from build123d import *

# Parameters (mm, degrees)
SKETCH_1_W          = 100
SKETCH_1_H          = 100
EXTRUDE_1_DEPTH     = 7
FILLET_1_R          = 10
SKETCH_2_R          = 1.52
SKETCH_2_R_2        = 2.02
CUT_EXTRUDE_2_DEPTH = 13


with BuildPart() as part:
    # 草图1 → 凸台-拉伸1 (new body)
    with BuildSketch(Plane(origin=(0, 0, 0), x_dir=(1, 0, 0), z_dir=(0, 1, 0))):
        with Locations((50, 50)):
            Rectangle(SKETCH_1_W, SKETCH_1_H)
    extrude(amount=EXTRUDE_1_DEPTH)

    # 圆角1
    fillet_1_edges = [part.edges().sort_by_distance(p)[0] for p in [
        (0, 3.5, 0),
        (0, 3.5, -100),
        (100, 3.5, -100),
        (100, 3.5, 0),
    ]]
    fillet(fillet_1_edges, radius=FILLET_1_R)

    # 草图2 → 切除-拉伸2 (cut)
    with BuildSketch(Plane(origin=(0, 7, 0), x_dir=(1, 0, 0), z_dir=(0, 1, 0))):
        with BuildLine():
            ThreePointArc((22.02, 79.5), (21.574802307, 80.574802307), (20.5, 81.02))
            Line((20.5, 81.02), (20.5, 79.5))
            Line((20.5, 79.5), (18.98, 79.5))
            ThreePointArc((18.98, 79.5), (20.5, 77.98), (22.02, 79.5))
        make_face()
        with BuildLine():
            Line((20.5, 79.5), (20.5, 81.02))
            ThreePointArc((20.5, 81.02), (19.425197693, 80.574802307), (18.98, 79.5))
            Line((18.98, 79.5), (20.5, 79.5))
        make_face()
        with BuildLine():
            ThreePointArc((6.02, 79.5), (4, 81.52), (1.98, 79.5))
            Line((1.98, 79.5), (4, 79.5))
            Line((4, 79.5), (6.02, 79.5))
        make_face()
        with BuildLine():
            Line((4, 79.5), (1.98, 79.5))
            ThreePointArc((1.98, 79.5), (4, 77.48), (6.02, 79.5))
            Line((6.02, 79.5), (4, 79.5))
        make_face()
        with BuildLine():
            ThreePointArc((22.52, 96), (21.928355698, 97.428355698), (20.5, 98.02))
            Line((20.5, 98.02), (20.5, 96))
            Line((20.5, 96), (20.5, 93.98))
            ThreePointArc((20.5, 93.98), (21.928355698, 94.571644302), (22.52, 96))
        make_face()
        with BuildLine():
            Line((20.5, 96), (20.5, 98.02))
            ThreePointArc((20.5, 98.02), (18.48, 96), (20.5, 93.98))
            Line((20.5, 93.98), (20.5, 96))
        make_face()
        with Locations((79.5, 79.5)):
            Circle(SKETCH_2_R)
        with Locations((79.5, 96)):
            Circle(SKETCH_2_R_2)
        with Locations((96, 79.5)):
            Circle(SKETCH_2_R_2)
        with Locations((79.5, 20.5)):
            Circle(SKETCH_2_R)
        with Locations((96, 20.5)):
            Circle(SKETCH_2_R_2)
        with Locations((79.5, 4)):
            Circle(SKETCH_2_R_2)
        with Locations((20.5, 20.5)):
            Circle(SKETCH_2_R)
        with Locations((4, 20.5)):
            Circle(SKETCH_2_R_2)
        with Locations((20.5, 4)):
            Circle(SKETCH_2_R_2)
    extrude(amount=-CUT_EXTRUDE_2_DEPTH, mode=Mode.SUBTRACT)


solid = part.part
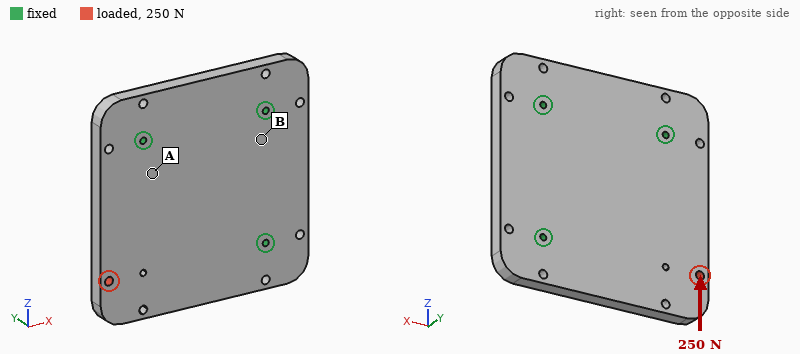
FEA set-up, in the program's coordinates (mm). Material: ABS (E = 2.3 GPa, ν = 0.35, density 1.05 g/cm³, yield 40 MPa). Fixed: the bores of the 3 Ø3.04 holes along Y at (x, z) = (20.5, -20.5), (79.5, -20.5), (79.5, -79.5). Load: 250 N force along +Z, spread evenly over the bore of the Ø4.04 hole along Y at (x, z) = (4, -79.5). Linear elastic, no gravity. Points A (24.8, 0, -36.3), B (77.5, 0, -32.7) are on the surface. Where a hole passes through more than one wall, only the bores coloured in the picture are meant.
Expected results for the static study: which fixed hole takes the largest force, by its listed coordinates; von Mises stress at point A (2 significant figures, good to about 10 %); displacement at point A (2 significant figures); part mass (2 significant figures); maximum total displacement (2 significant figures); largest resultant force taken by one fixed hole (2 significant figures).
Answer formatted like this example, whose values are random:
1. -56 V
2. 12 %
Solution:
1. (20.5, -20.5)
2. 0.95 MPa
3. 11 µm
4. 72 g
5. 58 µm
6. 230 N
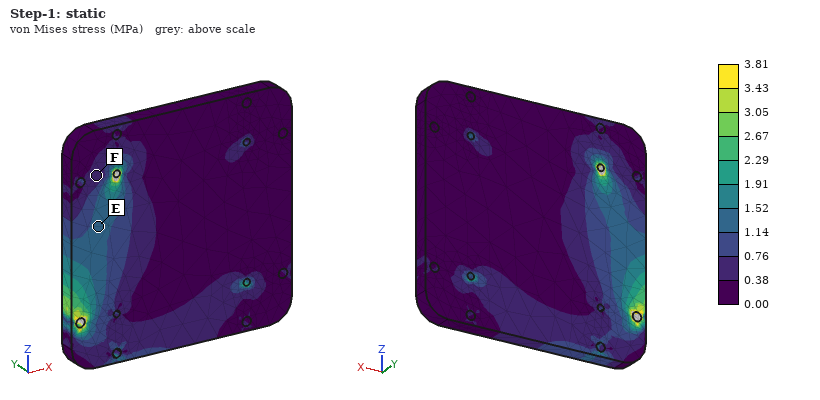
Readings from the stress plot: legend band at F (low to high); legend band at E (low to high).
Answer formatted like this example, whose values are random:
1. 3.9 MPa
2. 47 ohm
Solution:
1. 0.38 to 0.76 MPa
2. 1.14 to 1.52 MPa
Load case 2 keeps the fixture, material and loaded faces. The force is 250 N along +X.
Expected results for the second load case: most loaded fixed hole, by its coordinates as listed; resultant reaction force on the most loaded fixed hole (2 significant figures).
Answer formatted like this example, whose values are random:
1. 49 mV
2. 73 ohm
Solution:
1. (79.5, -79.5)
2. 190 N
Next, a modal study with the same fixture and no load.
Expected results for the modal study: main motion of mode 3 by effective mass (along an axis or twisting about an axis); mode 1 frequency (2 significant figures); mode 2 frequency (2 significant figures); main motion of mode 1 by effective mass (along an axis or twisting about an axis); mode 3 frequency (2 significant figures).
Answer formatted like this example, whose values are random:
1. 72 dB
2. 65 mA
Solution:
1. along Y
2. 460 Hz
3. 1400 Hz
4. along Y
5. 1600 Hz
